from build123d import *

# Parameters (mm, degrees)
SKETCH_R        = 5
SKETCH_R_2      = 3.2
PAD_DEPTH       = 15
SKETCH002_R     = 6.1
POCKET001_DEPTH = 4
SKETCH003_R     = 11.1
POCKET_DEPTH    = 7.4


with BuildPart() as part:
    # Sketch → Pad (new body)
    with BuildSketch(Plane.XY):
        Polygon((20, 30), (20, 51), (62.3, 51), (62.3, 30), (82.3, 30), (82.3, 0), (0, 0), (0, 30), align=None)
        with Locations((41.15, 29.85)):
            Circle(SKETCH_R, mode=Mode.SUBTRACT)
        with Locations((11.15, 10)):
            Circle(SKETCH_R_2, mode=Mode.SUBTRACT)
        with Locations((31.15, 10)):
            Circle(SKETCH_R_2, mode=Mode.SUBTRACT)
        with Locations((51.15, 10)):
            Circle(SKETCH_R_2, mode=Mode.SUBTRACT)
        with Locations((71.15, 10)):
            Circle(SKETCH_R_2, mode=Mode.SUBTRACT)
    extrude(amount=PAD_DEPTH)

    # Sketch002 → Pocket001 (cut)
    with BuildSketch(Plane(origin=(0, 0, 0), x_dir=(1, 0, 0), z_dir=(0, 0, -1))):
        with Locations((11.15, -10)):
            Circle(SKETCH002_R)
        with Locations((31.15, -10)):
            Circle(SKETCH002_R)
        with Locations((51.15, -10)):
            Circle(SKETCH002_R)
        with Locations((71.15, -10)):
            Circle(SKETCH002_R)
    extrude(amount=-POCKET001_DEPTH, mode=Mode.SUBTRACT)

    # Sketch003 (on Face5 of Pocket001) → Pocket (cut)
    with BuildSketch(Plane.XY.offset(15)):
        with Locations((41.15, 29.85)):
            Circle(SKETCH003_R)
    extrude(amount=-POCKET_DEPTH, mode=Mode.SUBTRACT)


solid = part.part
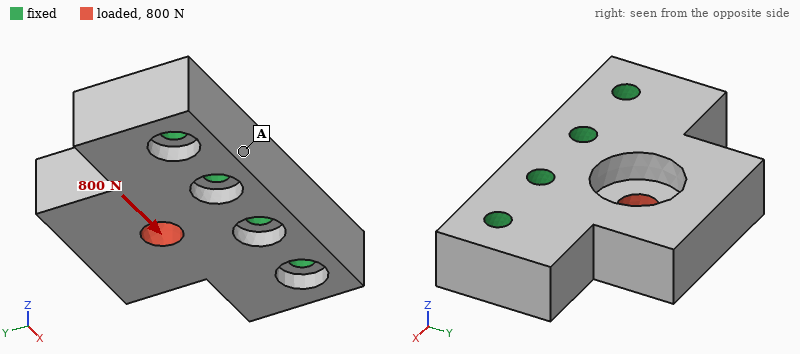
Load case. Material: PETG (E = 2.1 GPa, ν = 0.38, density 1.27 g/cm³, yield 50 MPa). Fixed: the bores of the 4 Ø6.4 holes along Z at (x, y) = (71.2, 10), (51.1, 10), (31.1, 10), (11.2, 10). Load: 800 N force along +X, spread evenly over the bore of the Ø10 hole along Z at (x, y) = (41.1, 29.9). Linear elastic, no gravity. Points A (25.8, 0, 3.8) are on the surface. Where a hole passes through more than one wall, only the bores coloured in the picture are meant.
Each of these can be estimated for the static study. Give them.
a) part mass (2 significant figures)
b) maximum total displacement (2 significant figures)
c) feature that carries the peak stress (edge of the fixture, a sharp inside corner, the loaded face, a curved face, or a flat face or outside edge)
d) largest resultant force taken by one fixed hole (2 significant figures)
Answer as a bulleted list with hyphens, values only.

- 55 g
- 53 µm
- the loaded face
- 300 N
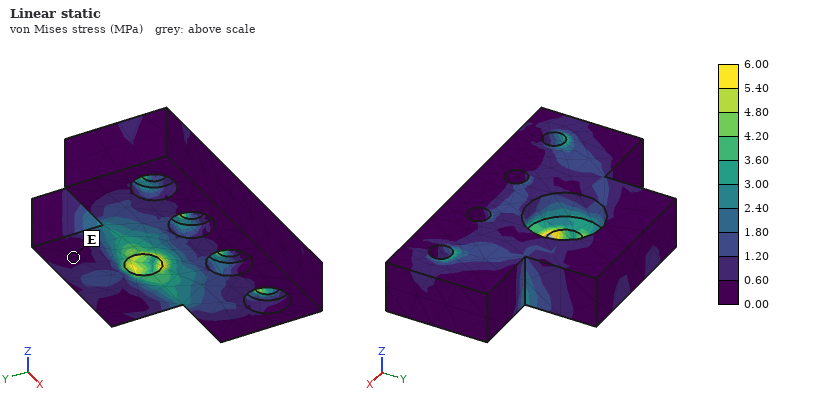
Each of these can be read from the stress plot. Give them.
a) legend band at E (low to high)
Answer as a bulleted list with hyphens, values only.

- 0.00 to 0.60 MPa
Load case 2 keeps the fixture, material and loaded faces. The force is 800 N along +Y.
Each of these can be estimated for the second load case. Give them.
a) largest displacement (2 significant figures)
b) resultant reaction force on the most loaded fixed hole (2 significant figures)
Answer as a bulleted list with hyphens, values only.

- 99 µm
- 310 N
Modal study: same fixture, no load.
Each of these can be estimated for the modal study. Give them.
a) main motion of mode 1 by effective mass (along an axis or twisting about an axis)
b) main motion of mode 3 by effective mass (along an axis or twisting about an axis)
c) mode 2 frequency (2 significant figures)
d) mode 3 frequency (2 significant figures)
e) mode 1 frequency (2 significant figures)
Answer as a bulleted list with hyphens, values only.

- along Z
- along X
- 3100 Hz
- 4200 Hz
- 1600 Hz
